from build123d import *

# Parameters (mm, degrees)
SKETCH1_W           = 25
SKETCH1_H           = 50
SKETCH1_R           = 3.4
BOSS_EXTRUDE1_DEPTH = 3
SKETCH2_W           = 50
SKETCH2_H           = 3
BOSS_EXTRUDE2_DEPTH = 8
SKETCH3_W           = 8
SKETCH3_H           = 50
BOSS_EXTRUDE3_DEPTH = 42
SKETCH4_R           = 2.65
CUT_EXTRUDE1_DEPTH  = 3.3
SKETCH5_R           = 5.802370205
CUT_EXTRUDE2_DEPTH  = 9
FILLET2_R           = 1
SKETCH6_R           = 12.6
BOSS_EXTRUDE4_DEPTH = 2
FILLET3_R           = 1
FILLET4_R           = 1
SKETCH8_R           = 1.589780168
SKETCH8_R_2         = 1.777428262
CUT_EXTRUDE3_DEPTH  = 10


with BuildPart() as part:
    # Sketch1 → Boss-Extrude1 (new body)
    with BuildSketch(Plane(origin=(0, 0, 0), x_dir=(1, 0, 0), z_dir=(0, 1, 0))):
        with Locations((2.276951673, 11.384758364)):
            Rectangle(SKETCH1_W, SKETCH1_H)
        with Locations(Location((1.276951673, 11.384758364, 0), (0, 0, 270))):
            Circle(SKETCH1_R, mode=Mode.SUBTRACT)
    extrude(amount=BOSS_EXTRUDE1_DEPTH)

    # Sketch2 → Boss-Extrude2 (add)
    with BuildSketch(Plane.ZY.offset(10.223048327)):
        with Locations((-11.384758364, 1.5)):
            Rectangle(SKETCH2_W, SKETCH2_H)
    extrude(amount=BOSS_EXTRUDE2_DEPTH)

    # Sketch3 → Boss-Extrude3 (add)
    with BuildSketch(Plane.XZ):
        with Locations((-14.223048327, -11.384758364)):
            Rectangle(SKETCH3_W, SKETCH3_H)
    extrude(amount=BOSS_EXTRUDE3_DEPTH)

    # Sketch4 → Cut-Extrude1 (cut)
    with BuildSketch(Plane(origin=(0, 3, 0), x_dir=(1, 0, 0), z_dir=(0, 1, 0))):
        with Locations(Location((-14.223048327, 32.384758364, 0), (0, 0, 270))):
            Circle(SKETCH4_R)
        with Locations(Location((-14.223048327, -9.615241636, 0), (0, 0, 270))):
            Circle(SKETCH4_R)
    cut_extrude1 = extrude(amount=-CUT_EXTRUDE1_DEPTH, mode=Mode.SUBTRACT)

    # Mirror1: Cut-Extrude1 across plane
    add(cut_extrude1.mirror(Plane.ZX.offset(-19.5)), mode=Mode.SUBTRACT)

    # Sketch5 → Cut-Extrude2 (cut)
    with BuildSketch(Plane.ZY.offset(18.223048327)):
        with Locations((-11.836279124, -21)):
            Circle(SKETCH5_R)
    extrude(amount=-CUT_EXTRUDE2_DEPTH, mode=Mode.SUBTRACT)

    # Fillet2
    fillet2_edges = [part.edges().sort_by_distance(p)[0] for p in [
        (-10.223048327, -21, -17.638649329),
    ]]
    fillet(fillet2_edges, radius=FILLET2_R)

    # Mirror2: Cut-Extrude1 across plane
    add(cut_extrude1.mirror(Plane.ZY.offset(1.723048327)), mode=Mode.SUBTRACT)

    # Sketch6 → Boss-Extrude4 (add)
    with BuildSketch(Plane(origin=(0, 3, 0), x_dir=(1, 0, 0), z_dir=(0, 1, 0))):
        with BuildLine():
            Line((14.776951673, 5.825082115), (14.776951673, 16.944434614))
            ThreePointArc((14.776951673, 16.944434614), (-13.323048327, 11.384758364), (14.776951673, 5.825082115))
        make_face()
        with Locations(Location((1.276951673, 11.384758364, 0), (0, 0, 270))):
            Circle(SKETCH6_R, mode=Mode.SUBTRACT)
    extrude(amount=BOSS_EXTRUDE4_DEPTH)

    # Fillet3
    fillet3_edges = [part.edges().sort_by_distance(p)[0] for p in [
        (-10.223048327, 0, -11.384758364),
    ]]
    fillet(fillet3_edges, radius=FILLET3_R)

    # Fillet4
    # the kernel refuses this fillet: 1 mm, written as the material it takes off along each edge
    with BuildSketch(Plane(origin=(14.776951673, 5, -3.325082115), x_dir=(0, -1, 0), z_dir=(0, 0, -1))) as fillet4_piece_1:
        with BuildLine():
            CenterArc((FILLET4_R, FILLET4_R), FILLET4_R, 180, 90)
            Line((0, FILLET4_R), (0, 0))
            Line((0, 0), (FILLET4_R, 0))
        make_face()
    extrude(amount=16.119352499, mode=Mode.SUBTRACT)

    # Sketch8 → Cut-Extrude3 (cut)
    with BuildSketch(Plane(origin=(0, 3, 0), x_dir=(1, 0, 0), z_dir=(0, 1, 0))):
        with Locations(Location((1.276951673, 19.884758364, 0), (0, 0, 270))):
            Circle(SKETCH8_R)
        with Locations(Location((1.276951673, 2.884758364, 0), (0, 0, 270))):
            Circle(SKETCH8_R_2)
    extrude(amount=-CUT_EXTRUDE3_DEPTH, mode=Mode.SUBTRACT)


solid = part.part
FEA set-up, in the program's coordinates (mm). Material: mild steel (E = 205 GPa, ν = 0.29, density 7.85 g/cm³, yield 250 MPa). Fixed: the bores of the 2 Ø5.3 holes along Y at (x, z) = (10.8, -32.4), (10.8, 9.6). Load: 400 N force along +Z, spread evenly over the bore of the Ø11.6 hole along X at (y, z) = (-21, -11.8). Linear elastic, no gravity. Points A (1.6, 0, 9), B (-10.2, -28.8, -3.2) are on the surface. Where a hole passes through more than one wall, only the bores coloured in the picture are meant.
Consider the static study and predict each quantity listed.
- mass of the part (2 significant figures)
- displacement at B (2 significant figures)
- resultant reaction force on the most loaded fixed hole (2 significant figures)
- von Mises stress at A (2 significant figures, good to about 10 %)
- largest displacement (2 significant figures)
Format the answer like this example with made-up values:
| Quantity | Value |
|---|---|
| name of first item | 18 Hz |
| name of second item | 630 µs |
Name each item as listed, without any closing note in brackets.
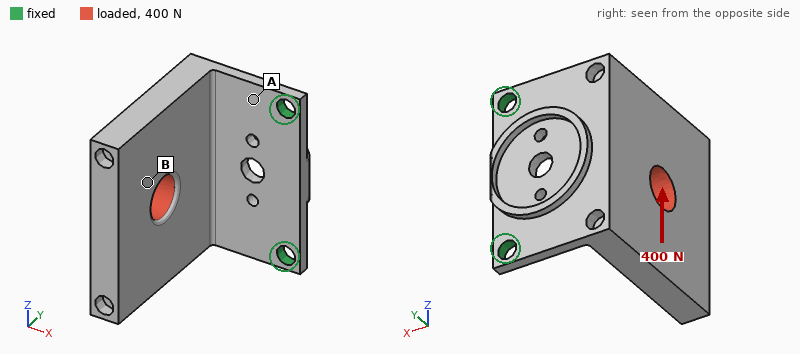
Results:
| Quantity | Value |
|---|---|
| mass of the part | 160 g |
| displacement at B | 39 µm |
| resultant reaction force on the most loaded fixed hole | 380 N |
| von Mises stress at A | 39 MPa |
| largest displacement | 61 µm |
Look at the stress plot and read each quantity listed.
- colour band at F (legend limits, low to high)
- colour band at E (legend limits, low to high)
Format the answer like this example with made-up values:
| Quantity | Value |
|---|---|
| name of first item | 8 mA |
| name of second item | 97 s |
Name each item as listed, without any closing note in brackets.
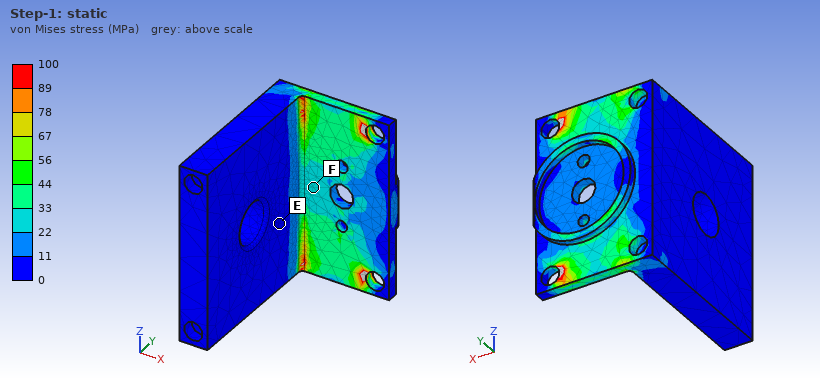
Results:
| Quantity | Value |
|---|---|
| colour band at F | 22 to 33 MPa |
| colour band at E | 0 to 11 MPa |
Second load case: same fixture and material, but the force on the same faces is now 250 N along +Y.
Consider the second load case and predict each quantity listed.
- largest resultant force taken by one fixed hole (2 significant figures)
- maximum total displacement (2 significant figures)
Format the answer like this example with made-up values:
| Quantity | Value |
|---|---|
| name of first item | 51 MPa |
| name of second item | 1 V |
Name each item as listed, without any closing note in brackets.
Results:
| Quantity | Value |
|---|---|
| largest resultant force taken by one fixed hole | 130 N |
| maximum total displacement | 0.17 mm |
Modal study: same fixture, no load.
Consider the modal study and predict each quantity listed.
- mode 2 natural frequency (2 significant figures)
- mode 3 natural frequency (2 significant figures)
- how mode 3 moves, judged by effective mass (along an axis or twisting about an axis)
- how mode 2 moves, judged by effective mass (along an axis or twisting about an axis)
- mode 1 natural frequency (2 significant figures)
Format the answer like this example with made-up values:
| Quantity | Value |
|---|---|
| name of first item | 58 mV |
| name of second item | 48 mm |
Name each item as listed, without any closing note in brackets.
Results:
| Quantity | Value |
|---|---|
| mode 2 natural frequency | 1300 Hz |
| mode 3 natural frequency | 2200 Hz |
| how mode 3 moves, judged by effective mass | along Y |
| how mode 2 moves, judged by effective mass | along Z |
| mode 1 natural frequency | 500 Hz |
